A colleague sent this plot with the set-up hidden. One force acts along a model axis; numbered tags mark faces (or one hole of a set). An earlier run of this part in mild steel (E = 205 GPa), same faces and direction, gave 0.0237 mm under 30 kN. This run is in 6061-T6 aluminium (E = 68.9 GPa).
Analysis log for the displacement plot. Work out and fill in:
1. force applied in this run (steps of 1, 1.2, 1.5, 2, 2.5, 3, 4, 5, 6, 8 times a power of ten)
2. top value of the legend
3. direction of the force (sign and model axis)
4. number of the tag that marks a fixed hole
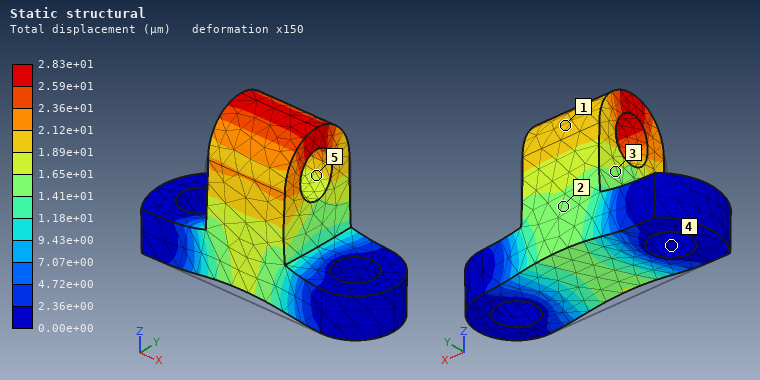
12 kN
2.83e+01 µm
+Z
4
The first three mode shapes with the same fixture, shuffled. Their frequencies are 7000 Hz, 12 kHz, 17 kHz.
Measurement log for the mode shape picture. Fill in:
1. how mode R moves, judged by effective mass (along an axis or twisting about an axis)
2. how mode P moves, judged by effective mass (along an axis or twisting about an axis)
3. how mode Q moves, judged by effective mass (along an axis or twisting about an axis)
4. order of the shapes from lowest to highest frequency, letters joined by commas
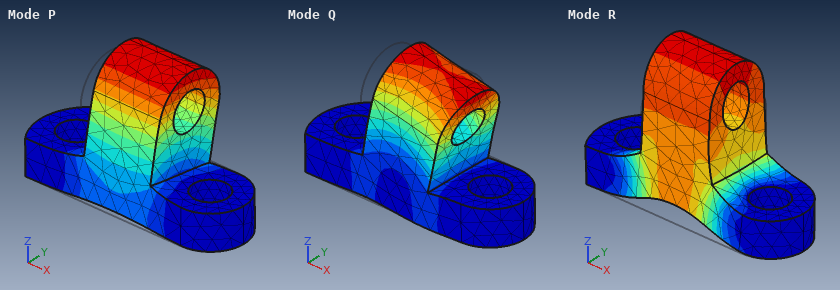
along Z
along Y
along X
P, Q, R
